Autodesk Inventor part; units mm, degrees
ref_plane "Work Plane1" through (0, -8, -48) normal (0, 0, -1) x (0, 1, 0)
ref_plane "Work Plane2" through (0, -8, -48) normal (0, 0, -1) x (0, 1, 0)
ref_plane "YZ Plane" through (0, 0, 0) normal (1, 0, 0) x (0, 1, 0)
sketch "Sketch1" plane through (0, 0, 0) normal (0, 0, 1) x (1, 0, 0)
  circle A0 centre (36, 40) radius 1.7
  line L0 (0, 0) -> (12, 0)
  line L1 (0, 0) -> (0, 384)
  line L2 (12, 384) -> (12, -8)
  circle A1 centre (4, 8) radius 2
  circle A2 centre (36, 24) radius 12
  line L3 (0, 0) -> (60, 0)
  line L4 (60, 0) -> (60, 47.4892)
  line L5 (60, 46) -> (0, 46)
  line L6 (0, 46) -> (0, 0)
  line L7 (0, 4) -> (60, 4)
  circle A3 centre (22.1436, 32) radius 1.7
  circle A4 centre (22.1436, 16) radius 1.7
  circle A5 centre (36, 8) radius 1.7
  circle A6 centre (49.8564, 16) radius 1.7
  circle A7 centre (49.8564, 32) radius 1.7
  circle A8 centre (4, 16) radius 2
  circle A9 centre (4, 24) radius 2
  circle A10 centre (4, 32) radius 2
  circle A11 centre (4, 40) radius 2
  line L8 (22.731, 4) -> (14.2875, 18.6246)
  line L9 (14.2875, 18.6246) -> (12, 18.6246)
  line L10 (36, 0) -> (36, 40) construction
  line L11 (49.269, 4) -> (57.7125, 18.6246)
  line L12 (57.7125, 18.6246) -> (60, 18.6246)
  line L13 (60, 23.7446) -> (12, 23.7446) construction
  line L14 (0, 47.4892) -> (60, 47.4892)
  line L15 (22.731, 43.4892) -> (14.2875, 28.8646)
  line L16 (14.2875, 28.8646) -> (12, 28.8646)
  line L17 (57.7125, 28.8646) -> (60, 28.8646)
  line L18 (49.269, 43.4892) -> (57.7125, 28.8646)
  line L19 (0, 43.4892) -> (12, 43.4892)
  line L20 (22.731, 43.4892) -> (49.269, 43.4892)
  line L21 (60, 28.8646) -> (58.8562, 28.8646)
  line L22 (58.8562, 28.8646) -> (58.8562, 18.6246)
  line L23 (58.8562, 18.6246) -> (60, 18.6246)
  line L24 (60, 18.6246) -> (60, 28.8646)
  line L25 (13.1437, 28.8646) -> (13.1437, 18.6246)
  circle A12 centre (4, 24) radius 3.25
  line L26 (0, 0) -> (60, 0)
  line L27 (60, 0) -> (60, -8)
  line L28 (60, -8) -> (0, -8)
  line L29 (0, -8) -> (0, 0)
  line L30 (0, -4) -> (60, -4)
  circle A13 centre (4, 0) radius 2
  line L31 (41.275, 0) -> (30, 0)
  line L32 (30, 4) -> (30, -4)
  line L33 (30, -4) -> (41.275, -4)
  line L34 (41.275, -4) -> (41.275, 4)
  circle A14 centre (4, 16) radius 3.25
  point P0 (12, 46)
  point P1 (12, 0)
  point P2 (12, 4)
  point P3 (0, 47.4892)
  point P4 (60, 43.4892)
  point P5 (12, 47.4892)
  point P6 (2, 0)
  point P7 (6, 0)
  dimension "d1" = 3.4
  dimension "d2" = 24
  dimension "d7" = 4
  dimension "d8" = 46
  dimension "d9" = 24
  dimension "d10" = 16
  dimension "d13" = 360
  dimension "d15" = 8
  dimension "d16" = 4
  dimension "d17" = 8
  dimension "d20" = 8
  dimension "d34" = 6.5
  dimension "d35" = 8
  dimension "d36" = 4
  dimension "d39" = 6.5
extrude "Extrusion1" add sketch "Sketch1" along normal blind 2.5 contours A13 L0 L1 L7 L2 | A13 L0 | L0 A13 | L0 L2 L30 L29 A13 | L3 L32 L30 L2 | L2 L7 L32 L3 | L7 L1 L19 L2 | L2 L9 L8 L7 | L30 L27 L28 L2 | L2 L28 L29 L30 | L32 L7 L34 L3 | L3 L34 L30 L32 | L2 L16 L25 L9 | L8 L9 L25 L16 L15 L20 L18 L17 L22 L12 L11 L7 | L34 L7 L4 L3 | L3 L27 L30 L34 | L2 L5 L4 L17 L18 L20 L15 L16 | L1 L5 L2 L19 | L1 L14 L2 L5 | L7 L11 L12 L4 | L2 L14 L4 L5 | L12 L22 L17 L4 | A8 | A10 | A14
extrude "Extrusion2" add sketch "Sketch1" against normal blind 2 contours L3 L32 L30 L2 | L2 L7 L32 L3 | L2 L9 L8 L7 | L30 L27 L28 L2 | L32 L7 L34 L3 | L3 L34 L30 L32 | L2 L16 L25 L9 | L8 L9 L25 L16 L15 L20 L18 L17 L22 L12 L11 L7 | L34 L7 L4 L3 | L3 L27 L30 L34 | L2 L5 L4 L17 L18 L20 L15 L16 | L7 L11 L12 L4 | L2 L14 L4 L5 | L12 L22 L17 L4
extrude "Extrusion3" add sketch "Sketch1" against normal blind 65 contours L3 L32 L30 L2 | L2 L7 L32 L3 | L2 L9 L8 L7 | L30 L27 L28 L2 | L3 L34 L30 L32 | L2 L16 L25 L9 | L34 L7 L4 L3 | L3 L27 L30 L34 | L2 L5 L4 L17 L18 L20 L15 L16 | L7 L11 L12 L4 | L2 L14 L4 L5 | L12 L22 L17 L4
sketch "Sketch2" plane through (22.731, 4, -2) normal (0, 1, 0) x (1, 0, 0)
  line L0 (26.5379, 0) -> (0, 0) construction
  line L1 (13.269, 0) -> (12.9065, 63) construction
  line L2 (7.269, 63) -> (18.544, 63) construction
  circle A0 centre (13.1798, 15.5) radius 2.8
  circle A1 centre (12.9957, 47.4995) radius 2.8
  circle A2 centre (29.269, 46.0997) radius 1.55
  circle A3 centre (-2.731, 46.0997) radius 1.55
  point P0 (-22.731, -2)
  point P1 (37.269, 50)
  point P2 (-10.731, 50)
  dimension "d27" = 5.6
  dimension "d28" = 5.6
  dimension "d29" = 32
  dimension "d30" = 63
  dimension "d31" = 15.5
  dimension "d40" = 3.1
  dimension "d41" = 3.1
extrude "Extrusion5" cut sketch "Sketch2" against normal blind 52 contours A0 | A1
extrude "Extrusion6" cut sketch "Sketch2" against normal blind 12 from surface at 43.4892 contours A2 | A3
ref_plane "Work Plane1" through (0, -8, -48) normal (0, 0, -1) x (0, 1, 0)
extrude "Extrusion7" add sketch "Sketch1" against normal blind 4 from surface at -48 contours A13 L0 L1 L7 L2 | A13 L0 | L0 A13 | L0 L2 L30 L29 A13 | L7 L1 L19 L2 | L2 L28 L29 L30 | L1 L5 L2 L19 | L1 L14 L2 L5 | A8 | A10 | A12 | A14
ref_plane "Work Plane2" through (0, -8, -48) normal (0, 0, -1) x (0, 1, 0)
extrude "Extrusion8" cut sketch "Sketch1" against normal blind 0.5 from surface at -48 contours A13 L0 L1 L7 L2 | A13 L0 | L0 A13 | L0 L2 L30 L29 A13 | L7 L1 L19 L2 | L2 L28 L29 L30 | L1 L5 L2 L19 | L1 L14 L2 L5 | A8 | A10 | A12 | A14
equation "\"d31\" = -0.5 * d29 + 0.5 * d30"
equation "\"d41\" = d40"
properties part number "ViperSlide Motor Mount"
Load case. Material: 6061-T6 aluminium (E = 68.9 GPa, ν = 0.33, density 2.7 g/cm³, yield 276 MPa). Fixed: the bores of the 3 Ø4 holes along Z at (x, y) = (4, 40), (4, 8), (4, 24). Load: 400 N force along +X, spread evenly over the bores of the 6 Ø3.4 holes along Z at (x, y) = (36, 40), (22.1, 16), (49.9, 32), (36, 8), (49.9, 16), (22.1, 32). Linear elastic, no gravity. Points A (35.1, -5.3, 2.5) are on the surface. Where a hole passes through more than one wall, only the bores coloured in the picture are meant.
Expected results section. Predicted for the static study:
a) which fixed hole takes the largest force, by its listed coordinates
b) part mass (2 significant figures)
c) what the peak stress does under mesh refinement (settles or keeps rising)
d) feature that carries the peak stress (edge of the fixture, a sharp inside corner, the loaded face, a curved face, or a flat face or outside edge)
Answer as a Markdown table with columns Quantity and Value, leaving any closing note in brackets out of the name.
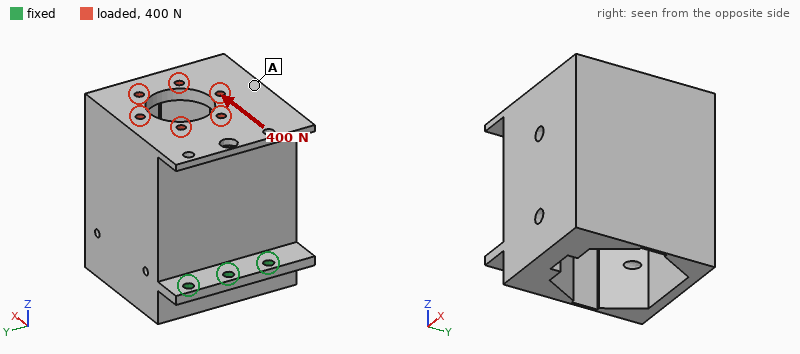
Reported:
| Quantity | Value |
|---|---|
| which fixed hole takes the largest force, by its listed coordinates | (4, 24) |
| part mass | 230 g |
| what the peak stress does under mesh refinement | keeps rising |
| feature that carries the peak stress | edge of the fixture |
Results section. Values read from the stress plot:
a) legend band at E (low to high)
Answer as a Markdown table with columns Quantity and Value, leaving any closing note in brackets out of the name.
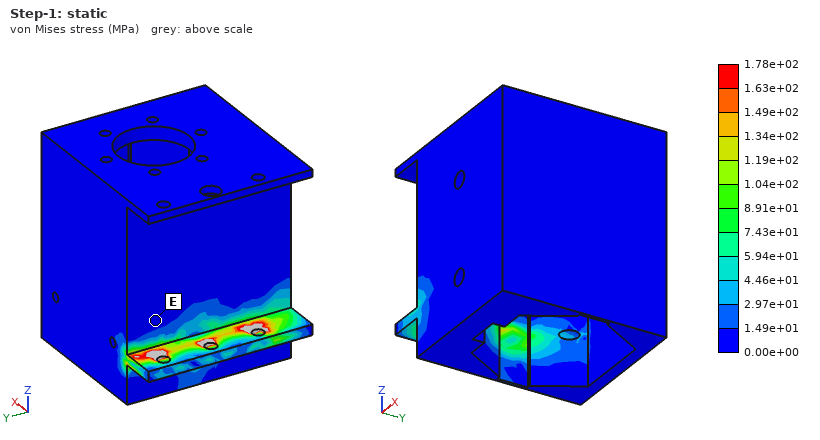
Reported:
| Quantity | Value |
|---|---|
| legend band at E | 0.00e+00 to 1.49e+01 MPa |
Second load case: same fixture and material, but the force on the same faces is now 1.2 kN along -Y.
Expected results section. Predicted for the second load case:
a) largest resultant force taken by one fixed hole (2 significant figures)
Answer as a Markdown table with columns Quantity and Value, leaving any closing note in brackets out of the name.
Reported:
| Quantity | Value |
|---|---|
| largest resultant force taken by one fixed hole | 2.1 kN |
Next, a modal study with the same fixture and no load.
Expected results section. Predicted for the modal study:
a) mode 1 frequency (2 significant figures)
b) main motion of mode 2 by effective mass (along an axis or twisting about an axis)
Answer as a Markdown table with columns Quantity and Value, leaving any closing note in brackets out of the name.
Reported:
| Quantity | Value |
|---|---|
| mode 1 frequency | 290 Hz |
| main motion of mode 2 by effective mass | along Y |
